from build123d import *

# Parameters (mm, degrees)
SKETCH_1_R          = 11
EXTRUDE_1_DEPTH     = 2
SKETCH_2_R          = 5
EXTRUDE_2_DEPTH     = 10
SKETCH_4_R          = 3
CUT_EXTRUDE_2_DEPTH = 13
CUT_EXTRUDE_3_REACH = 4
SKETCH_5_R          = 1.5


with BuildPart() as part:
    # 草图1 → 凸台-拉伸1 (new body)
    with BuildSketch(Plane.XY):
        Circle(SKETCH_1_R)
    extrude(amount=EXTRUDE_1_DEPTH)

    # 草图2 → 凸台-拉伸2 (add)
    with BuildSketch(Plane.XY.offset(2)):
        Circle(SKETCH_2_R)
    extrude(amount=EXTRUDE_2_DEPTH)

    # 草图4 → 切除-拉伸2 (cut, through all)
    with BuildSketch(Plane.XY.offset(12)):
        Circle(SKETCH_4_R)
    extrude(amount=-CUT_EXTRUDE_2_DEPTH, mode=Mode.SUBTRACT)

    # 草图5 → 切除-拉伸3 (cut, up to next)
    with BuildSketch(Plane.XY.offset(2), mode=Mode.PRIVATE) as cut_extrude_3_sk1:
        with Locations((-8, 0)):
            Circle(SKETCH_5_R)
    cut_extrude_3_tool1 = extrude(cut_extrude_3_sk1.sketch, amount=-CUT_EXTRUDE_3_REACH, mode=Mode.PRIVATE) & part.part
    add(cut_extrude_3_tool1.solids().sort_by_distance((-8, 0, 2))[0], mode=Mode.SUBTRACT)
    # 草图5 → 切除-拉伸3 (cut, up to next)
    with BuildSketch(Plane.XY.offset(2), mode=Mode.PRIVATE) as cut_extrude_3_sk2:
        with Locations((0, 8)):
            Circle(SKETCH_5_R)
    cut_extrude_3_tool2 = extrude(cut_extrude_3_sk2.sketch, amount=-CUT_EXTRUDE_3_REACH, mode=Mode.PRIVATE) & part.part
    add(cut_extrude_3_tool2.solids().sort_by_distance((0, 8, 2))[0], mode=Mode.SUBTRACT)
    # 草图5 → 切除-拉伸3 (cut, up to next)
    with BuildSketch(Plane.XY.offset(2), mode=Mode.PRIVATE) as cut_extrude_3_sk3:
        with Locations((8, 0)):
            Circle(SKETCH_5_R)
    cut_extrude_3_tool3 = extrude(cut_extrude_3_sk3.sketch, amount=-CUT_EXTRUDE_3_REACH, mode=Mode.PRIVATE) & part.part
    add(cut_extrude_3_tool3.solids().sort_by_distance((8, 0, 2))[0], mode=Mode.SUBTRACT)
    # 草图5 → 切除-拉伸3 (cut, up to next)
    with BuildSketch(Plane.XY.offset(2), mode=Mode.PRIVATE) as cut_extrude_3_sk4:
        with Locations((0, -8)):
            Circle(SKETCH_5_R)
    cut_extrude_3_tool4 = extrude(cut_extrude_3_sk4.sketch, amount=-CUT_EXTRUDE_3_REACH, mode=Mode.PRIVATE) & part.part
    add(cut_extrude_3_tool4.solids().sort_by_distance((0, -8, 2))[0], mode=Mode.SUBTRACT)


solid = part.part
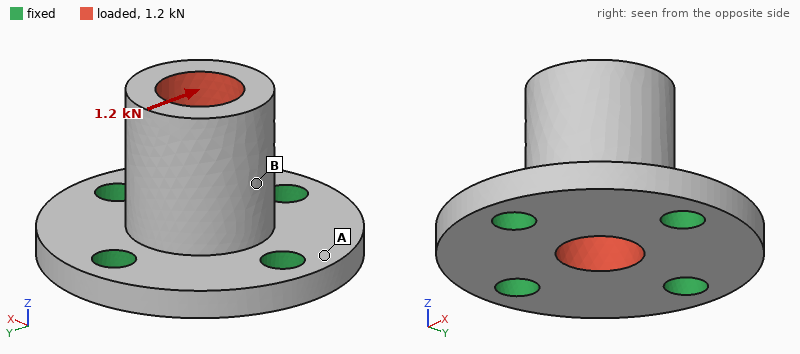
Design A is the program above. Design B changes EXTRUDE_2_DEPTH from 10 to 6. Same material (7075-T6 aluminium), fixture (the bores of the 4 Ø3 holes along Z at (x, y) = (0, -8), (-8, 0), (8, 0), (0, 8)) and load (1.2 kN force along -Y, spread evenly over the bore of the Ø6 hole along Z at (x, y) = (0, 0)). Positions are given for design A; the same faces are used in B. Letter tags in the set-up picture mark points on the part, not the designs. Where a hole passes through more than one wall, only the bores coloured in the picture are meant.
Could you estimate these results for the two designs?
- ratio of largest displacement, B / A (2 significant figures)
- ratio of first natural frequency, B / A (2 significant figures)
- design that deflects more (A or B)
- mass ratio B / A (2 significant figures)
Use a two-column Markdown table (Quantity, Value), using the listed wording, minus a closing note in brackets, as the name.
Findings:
| Quantity | Value |
|---|---|
| ratio of largest displacement, B / A | 0.44 |
| ratio of first natural frequency, B / A | 1.8 |
| design that deflects more | A |
| mass ratio B / A | 0.83 |
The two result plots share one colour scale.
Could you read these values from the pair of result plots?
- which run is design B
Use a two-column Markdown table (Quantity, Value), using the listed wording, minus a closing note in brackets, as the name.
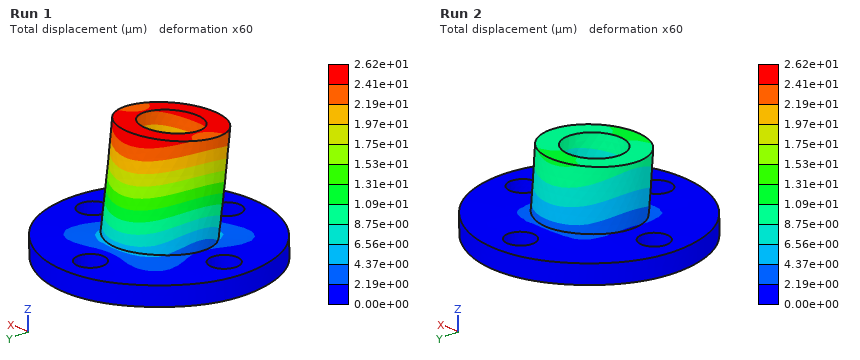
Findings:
| Quantity | Value |
|---|---|
| which run is design B | Run 2 |
